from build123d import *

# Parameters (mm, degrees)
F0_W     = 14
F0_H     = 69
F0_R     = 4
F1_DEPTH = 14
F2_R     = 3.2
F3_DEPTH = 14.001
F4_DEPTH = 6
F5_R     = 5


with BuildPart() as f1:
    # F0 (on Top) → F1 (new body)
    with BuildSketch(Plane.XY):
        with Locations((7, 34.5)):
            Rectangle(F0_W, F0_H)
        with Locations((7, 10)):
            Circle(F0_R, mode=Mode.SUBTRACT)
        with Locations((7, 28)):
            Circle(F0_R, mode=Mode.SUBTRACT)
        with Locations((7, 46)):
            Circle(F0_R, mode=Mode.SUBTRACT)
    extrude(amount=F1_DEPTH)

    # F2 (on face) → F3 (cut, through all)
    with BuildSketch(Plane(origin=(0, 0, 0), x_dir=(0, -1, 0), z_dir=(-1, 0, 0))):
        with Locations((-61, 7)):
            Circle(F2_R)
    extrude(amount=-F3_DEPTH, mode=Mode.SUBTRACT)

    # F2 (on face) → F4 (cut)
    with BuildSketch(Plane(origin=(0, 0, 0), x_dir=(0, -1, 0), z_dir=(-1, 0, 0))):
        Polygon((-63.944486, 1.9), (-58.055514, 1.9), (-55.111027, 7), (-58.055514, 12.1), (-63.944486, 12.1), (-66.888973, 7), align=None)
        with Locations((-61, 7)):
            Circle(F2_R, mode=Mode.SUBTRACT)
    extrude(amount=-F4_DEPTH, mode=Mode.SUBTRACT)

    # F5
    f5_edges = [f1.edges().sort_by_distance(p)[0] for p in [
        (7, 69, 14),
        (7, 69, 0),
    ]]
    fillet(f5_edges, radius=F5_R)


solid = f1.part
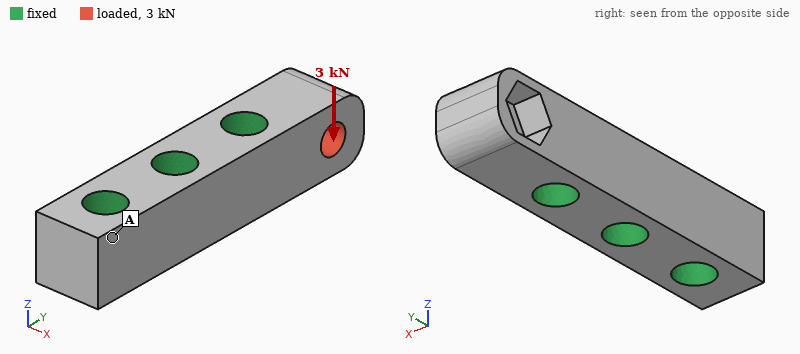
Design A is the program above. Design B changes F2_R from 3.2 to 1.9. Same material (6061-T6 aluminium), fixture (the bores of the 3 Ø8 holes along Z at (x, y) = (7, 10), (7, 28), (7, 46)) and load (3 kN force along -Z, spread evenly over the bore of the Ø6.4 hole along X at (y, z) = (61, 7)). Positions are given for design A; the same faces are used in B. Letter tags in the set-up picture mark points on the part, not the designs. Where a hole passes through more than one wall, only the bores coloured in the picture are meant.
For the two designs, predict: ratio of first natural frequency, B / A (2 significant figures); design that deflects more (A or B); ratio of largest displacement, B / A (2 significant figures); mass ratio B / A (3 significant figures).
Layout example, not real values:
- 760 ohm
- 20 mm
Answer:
- 1.0
- A
- 0.81
- 1.02
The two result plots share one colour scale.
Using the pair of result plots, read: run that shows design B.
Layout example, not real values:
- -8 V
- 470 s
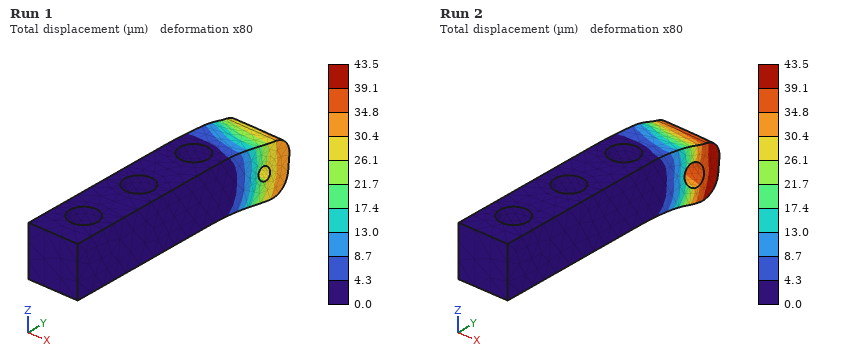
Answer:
- Run 1
